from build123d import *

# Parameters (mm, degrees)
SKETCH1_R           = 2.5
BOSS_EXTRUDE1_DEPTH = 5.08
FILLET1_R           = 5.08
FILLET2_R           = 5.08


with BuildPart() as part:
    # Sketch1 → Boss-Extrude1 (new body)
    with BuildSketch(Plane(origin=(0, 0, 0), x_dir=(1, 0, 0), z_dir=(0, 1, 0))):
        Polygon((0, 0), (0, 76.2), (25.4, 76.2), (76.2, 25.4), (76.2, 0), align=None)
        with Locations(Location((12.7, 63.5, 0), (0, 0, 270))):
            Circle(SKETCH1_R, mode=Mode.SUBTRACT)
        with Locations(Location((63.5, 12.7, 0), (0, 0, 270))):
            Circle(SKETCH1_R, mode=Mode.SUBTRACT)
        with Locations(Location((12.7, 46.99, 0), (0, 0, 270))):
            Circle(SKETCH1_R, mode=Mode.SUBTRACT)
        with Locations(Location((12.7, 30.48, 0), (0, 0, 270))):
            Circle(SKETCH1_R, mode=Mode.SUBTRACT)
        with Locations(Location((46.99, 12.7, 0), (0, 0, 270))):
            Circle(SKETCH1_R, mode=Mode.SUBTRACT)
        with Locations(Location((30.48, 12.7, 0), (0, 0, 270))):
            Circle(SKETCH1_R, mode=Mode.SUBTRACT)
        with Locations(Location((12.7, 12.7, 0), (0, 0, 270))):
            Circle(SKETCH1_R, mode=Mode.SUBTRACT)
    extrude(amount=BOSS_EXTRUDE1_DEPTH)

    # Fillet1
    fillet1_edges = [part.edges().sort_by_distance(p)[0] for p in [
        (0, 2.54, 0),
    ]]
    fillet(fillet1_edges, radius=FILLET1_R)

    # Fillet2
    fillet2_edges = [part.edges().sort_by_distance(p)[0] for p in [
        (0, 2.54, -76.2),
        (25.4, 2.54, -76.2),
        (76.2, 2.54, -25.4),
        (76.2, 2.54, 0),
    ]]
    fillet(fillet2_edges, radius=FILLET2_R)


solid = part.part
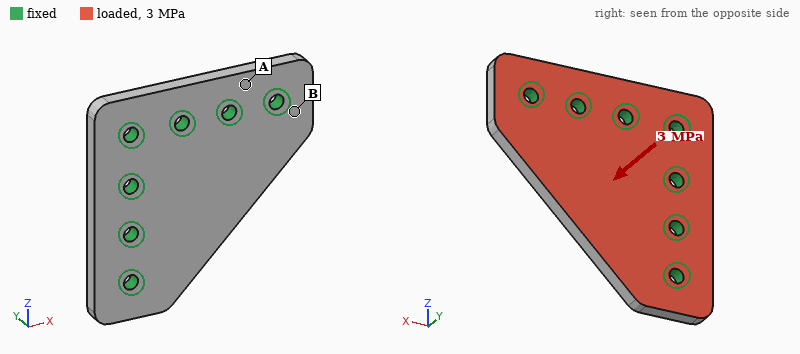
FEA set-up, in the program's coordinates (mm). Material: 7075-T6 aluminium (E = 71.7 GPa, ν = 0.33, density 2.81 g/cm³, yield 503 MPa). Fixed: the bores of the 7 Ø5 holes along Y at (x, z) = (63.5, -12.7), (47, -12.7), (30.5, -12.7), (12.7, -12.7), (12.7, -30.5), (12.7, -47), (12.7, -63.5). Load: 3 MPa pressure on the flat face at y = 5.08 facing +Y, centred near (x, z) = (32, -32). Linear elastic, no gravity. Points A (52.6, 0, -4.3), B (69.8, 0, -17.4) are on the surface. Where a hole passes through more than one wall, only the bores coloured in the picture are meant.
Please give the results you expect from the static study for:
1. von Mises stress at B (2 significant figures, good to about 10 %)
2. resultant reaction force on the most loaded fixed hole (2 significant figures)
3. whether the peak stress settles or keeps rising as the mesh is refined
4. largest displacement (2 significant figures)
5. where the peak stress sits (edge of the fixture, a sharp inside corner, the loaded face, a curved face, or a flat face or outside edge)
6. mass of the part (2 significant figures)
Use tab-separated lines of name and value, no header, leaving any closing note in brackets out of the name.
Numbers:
von Mises stress at B	110 MPa
resultant reaction force on the most loaded fixed hole	2.5 kN
whether the peak stress settles or keeps rising as the mesh is refined	keeps rising
largest displacement	0.28 mm
where the peak stress sits	edge of the fixture
mass of the part	62 g
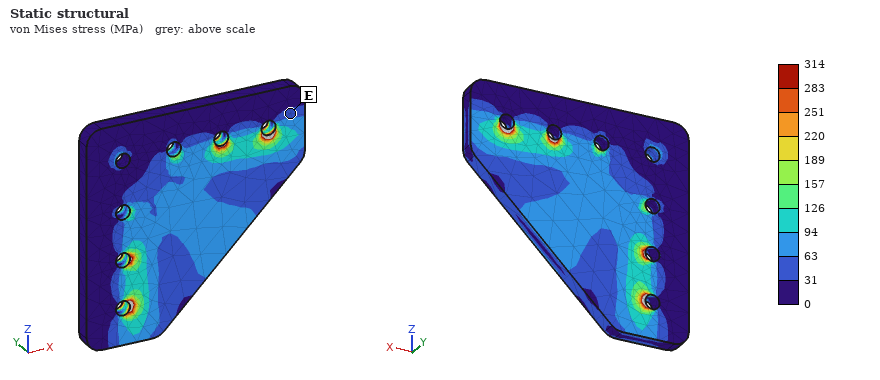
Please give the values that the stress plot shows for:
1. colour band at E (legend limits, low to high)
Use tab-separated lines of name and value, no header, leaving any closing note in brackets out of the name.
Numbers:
colour band at E	31 to 63 MPa
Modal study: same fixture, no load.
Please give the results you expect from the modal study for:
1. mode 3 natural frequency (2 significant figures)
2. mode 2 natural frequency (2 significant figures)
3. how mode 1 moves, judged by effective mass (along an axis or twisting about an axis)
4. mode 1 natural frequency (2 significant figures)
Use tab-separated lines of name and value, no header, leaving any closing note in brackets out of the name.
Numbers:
mode 3 natural frequency	16 kHz
mode 2 natural frequency	12 kHz
how mode 1 moves, judged by effective mass	along Y
mode 1 natural frequency	5900 Hz
